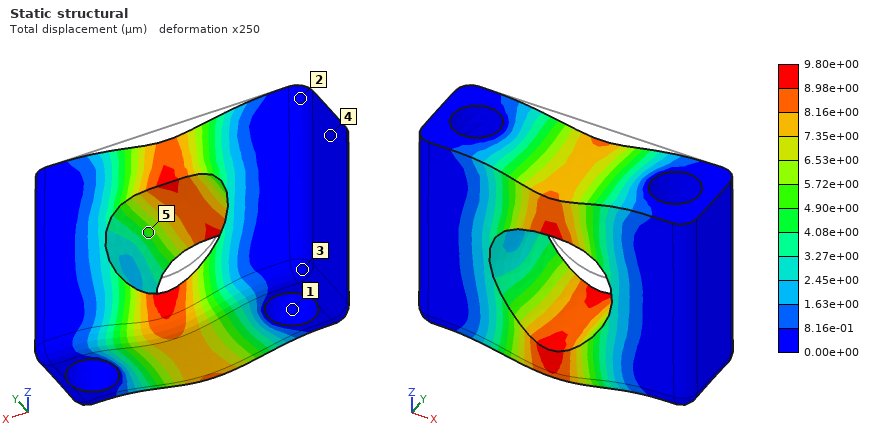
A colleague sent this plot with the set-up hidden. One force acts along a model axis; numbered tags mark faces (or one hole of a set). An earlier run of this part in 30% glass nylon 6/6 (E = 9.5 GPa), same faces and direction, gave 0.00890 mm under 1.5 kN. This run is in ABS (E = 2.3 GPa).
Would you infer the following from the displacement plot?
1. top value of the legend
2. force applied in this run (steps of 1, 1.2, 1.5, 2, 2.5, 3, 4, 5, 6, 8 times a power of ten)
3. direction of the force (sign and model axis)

9.80e+00 µm
400 N
-Z
